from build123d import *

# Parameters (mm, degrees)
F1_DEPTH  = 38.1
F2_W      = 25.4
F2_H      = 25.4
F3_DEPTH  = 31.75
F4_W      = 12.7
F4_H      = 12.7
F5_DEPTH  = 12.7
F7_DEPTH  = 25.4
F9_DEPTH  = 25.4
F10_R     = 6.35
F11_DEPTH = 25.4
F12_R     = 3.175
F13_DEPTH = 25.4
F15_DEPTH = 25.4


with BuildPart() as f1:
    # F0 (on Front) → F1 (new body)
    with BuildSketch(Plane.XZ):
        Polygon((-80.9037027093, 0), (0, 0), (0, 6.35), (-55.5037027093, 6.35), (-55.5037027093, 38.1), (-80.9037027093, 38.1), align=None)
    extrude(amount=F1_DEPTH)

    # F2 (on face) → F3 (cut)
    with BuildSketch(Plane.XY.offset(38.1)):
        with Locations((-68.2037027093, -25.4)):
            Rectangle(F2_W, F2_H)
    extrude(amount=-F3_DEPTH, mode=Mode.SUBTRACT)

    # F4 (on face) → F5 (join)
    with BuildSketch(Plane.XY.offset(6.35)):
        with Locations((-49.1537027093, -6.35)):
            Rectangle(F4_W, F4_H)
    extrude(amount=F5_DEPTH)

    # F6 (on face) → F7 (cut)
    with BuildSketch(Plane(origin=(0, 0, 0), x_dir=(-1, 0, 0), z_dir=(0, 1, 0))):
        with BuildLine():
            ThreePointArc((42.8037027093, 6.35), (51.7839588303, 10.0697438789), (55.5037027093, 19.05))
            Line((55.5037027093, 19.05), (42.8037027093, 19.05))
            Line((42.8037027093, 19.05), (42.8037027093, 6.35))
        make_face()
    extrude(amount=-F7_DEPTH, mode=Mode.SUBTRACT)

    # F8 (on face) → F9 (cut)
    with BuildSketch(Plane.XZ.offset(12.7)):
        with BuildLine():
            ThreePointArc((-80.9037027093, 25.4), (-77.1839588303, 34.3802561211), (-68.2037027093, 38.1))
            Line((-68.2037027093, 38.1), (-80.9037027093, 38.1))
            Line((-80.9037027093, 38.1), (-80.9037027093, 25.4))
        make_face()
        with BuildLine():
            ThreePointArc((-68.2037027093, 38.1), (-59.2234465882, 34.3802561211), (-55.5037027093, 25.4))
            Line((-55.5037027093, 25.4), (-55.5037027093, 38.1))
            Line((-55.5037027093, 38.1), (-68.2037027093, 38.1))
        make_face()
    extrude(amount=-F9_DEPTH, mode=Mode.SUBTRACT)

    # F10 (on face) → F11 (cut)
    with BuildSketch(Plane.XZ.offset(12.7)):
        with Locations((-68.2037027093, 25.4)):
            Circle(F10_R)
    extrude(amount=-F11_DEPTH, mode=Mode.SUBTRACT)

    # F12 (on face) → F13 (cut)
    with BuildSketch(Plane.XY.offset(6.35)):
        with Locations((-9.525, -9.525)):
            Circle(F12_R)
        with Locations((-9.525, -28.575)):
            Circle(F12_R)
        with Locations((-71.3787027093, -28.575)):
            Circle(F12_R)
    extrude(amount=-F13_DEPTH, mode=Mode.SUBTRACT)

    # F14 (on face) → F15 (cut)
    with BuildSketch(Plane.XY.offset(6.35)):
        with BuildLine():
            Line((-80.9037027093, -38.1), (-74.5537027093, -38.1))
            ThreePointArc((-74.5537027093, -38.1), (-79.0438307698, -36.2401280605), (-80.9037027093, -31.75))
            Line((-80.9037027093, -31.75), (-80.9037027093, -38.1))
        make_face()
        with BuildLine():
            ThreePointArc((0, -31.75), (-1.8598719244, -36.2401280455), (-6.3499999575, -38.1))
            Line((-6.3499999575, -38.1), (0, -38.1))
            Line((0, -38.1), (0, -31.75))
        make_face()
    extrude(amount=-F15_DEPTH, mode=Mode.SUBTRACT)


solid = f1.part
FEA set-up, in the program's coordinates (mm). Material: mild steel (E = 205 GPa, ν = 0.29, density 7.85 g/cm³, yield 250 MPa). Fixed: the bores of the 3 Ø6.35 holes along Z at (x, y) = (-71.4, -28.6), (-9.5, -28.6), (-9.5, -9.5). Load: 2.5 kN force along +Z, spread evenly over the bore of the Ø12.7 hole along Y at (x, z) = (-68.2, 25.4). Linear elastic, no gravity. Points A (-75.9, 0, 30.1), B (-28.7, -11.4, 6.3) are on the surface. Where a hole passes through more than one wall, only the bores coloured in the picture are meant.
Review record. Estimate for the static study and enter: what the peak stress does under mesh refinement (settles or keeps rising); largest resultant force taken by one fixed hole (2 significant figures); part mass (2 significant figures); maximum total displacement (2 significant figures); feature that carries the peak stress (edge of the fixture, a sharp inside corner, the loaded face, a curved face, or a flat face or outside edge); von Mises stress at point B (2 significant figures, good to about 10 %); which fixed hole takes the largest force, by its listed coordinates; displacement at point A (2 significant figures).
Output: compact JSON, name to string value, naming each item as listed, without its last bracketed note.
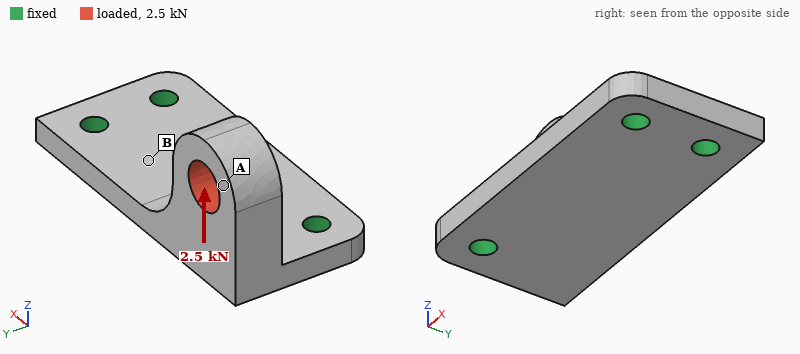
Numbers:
{"what the peak stress does under mesh refinement": "keeps rising", "largest resultant force taken by one fixed hole": "2.2 kN", "part mass": "210 g", "maximum total displacement": "0.12 mm", "feature that carries the peak stress": "edge of the fixture", "von Mises stress at point B": "52 MPa", "which fixed hole takes the largest force, by its listed coordinates": "(-71.4, -28.6)", "displacement at point A": "0.10 mm"}
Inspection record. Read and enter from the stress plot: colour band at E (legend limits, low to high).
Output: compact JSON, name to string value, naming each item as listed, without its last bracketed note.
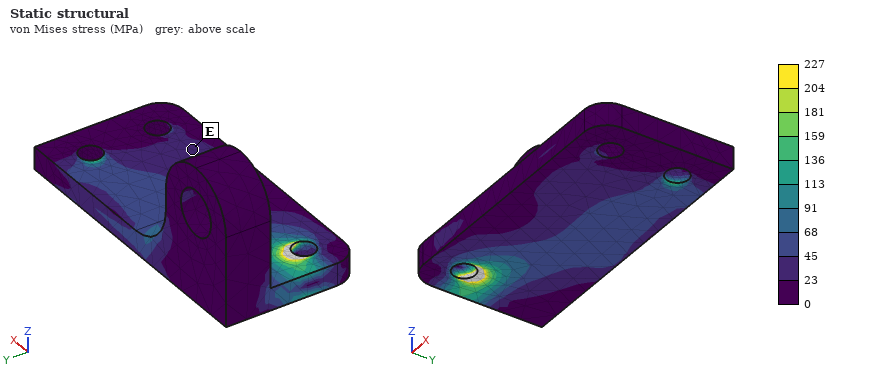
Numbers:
{"colour band at E": "23 to 45 MPa"}
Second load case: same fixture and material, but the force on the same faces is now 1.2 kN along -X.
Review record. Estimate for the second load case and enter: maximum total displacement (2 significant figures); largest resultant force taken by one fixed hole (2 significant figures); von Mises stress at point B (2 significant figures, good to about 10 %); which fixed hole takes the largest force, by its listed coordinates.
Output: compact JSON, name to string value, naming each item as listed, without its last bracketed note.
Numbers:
{"maximum total displacement": "32 µm", "largest resultant force taken by one fixed hole": "690 N", "von Mises stress at point B": "9.1 MPa", "which fixed hole takes the largest force, by its listed coordinates": "(-71.4, -28.6)"}
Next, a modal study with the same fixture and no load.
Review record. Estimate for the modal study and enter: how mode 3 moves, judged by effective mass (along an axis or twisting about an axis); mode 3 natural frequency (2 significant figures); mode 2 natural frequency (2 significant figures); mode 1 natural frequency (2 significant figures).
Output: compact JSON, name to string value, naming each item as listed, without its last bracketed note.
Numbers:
{"how mode 3 moves, judged by effective mass": "along Z", "mode 3 natural frequency": "7800 Hz", "mode 2 natural frequency": "4900 Hz", "mode 1 natural frequency": "2600 Hz"}
